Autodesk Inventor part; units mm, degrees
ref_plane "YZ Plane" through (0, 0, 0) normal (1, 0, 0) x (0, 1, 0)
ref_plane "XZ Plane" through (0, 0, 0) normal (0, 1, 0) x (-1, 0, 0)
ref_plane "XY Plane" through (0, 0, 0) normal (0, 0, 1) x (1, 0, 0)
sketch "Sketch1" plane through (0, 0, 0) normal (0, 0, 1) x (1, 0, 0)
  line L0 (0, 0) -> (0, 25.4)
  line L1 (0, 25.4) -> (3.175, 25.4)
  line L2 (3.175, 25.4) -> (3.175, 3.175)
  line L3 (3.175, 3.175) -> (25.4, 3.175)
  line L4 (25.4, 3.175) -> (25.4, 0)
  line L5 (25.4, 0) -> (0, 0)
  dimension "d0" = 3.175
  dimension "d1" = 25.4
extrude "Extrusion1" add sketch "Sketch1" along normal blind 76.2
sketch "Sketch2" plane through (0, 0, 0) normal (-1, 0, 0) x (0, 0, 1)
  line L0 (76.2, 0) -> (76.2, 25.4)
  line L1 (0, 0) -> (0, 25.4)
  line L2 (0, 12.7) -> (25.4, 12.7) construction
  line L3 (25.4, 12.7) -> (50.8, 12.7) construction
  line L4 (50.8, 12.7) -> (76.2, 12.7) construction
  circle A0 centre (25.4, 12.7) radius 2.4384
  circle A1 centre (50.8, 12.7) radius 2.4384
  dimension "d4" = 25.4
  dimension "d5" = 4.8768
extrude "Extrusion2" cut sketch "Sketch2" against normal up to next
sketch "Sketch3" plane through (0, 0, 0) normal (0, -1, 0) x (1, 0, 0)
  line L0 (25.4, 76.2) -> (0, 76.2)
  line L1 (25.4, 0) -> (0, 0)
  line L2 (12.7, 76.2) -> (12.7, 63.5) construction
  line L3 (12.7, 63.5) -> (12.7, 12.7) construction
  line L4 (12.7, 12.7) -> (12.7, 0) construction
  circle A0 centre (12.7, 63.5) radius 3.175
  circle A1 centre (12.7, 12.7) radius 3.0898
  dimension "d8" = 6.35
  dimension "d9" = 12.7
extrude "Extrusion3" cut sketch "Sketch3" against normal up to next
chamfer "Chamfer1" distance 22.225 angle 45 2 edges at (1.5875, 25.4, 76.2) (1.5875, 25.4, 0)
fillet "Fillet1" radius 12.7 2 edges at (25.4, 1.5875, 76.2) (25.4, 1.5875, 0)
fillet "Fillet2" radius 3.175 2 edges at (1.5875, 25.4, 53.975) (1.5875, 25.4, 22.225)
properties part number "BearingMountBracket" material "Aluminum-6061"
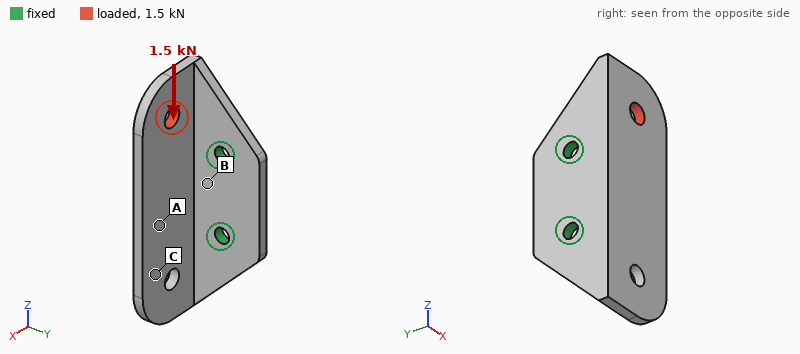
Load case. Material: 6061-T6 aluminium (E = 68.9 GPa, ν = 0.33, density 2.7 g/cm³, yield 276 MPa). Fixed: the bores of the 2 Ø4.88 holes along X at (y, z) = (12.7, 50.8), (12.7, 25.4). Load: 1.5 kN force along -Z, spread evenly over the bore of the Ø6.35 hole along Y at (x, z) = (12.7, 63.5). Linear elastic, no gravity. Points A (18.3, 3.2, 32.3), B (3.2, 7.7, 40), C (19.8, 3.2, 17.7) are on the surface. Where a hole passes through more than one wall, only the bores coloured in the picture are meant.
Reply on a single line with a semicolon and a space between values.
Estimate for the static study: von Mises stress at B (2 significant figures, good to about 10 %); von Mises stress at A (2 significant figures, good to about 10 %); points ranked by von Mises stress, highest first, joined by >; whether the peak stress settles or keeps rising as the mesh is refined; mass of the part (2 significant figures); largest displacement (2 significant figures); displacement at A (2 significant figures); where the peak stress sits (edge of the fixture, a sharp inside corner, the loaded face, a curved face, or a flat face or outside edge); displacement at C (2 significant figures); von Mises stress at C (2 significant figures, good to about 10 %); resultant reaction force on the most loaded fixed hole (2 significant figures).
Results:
49 MPa; 24 MPa; B > A > C; keeps rising; 25 g; 0.12 mm; 0.054 mm; edge of the fixture; 0.082 mm; 15 MPa; 1.1 kN
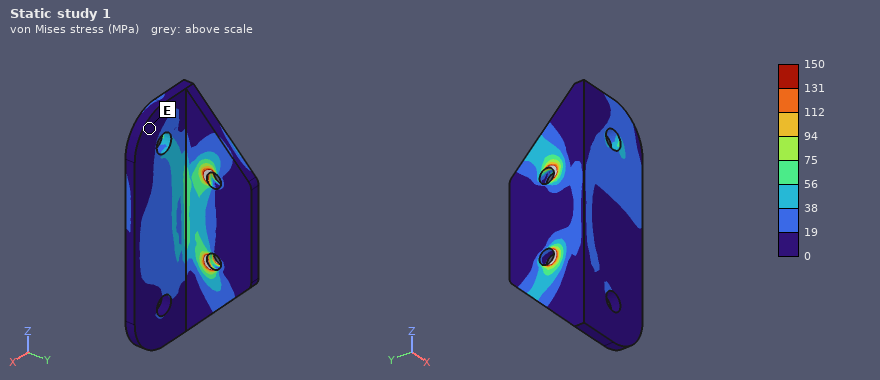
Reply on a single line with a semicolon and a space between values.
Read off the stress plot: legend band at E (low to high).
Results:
0 to 19 MPa
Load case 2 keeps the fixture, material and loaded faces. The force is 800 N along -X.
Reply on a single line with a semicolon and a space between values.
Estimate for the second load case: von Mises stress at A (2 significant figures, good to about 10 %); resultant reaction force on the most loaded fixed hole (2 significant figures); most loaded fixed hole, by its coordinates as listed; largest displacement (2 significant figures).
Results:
27 MPa; 1.1 kN; (12.7, 50.8); 0.25 mm
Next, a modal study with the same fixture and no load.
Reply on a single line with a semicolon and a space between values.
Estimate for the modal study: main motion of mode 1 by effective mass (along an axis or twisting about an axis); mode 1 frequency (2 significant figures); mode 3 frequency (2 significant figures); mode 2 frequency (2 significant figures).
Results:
along Y; 2600 Hz; 5600 Hz; 3300 Hz
